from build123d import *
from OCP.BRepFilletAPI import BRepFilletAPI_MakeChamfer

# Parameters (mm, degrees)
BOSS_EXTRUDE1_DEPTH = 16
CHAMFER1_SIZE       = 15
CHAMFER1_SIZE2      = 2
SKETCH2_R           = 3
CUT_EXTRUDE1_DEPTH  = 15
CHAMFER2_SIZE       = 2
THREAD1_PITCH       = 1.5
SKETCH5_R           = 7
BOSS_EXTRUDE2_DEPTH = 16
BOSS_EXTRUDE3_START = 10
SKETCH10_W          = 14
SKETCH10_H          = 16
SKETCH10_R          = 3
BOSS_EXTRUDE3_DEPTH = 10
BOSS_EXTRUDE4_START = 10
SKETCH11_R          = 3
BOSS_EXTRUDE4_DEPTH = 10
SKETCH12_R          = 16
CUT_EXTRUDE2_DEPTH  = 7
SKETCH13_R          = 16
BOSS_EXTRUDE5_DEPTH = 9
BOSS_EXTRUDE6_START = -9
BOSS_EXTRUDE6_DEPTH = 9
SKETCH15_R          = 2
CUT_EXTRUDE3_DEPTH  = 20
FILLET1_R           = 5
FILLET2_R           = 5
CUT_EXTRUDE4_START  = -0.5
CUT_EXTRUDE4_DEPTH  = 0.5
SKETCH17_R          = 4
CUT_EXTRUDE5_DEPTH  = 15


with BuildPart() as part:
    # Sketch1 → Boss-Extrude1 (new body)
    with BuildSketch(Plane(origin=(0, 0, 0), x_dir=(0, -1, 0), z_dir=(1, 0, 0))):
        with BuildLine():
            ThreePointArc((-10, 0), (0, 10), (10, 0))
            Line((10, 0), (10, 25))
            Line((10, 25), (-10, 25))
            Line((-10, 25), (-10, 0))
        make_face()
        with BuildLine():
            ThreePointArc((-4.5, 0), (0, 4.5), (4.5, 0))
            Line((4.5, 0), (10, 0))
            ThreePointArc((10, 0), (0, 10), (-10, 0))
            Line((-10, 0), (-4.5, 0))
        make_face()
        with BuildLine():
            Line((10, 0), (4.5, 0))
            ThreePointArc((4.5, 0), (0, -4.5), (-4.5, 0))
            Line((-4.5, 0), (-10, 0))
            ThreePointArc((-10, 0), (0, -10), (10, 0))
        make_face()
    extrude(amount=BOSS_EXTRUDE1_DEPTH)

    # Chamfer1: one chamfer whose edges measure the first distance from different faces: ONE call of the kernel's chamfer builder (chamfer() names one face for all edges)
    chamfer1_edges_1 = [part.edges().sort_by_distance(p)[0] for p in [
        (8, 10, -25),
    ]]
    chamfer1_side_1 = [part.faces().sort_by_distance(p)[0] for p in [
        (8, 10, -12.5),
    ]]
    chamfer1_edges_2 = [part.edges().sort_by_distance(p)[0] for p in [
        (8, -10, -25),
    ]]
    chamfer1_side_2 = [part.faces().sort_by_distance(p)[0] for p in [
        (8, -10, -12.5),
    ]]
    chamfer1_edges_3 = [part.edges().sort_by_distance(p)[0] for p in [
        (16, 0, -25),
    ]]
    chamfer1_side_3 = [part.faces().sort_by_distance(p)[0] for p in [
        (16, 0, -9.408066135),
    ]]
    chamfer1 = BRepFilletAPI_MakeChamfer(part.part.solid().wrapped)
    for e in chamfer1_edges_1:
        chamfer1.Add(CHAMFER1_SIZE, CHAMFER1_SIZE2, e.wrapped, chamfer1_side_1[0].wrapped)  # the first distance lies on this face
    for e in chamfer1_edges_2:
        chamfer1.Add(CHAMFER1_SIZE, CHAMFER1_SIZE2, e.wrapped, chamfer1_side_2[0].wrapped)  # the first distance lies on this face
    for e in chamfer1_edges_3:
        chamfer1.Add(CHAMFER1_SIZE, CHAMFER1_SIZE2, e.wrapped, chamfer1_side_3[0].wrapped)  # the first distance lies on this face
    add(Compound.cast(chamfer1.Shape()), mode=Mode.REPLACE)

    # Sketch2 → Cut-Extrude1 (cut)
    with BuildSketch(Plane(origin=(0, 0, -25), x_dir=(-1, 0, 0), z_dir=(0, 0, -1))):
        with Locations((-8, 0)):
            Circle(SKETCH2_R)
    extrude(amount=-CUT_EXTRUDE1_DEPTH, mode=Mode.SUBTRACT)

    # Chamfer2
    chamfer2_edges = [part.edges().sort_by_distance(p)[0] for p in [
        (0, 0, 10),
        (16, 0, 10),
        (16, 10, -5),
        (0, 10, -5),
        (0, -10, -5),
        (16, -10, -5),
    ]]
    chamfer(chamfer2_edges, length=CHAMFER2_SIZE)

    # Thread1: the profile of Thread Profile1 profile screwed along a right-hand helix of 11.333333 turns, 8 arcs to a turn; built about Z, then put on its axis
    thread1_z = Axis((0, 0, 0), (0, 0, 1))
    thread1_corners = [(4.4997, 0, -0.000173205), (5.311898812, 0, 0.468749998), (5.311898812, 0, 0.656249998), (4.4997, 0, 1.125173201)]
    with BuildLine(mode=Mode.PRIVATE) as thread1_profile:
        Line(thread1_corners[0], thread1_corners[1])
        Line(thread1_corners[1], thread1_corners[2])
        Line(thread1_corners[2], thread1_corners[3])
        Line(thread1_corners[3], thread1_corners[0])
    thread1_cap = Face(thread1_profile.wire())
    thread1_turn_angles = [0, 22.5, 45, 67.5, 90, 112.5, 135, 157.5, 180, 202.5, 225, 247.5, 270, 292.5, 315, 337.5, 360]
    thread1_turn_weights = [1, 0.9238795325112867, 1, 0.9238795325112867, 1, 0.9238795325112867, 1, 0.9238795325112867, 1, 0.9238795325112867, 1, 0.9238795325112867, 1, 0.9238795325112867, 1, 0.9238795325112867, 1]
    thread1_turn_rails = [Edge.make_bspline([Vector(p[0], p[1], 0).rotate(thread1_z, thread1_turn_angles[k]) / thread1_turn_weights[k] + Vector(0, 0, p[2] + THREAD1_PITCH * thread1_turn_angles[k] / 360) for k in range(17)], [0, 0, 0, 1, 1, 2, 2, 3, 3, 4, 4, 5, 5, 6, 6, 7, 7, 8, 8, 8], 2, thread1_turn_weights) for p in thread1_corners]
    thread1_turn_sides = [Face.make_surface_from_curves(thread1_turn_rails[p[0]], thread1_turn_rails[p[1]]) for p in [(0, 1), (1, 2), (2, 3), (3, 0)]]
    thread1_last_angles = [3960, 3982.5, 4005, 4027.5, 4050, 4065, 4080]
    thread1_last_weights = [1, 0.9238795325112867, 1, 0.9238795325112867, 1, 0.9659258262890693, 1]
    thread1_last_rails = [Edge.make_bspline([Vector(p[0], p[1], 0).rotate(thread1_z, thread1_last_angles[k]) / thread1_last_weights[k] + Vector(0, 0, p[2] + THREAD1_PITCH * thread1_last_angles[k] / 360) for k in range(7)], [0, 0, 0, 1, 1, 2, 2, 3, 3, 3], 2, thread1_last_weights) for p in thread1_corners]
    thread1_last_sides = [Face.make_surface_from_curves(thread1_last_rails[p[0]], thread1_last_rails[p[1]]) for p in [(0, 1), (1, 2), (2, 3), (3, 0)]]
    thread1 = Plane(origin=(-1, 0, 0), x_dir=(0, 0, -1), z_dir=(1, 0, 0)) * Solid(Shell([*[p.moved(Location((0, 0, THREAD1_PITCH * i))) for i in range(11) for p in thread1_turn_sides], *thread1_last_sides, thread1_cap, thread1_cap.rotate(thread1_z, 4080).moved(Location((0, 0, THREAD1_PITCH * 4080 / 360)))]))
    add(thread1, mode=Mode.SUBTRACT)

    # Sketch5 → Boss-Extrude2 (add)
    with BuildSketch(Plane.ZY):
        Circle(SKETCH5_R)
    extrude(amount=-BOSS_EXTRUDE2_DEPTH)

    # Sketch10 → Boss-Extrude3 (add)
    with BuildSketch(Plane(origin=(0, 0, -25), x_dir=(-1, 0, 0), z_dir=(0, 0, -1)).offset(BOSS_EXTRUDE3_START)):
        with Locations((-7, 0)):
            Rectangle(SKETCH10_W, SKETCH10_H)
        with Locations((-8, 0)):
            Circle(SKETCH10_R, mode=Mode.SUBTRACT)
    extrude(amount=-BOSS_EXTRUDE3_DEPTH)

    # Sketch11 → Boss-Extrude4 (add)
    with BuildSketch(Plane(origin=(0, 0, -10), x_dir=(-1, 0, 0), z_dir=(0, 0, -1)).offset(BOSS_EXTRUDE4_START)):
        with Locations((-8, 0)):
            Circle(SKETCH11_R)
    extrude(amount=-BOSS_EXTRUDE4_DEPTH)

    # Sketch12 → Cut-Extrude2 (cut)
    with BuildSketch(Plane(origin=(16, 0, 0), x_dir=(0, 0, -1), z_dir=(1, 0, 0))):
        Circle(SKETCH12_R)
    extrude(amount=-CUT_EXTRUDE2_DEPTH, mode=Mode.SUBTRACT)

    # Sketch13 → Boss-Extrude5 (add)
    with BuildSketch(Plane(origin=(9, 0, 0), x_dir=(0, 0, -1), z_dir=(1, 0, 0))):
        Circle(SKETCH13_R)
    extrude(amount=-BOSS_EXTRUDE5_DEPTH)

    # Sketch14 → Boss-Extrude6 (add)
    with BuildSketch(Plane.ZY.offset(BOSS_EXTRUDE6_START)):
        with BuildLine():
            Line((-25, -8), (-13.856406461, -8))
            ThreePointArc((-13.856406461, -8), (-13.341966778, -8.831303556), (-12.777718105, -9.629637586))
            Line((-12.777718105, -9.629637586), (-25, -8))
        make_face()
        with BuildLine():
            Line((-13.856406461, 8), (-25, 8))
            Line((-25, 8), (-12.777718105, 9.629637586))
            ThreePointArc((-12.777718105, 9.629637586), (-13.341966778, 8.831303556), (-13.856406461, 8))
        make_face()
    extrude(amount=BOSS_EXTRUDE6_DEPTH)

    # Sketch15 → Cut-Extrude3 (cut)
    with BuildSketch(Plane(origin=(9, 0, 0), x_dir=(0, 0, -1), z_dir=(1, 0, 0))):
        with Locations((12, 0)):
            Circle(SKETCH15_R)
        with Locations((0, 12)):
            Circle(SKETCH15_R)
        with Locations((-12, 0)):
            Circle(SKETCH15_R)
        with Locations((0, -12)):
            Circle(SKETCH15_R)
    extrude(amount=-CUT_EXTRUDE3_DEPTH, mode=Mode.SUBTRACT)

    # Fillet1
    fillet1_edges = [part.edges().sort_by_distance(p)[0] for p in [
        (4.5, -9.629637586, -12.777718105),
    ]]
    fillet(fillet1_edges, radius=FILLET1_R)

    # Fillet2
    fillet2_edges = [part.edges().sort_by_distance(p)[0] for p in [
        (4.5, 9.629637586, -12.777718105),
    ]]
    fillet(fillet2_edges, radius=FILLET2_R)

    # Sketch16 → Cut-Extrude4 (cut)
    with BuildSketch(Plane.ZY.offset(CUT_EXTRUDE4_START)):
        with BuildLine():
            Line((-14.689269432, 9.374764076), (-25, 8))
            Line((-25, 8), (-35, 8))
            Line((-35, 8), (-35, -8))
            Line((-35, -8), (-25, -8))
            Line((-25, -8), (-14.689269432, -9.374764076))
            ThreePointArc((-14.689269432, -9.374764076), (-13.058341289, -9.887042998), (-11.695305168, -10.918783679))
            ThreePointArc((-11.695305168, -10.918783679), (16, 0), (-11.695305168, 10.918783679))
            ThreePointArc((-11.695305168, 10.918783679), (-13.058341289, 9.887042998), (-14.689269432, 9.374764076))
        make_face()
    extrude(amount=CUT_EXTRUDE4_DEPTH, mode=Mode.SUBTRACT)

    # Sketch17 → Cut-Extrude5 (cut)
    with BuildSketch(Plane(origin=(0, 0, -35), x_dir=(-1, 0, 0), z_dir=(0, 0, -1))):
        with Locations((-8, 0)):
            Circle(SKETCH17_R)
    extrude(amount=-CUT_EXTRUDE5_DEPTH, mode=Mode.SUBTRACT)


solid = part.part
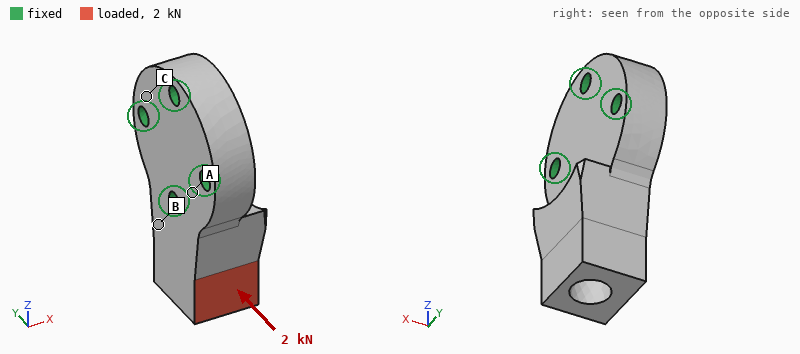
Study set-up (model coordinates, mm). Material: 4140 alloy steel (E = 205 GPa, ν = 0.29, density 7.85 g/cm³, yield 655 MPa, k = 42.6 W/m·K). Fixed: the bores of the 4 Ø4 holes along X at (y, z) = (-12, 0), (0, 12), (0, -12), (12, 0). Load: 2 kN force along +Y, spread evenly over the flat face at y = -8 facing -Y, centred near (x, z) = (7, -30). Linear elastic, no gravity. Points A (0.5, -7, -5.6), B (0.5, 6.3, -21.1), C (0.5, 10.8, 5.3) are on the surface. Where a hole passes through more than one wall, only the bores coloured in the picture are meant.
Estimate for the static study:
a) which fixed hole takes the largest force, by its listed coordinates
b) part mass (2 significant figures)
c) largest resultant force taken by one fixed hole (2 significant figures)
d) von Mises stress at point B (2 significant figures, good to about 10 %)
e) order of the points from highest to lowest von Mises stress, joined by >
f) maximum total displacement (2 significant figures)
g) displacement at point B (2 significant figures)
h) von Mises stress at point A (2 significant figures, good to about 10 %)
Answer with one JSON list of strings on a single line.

["(0, -12)", "81 g", "2.0 kN", "35 MPa", "B > A > C", "15 µm", "4.2 µm", "19 MPa"]
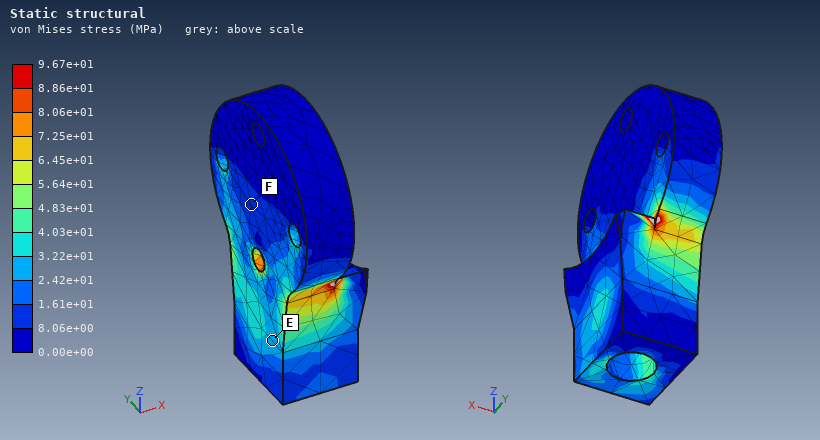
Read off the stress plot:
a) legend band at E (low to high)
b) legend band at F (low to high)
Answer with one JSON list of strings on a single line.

["2.42e+01 to 3.22e+01 MPa", "8.06e+00 to 1.61e+01 MPa"]
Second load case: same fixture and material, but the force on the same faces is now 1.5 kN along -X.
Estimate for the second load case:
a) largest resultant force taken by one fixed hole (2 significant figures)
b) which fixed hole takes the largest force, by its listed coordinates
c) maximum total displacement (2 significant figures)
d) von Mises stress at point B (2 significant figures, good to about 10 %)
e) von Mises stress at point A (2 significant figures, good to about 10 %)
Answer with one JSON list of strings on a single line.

["2.1 kN", "(0, -12)", "28 µm", "46 MPa", "22 MPa"]
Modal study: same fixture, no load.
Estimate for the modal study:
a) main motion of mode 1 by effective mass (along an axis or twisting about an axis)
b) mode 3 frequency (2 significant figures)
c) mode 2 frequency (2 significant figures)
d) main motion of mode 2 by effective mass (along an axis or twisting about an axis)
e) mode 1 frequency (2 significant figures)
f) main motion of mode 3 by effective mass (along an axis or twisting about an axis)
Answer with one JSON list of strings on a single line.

["along X", "24 kHz", "17 kHz", "along Y", "11 kHz", "twisting about Z"]
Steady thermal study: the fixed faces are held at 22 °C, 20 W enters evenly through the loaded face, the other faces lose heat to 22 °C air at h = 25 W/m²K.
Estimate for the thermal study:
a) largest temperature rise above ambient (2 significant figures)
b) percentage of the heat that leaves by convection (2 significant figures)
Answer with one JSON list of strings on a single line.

["71 K", "7.7 %"]
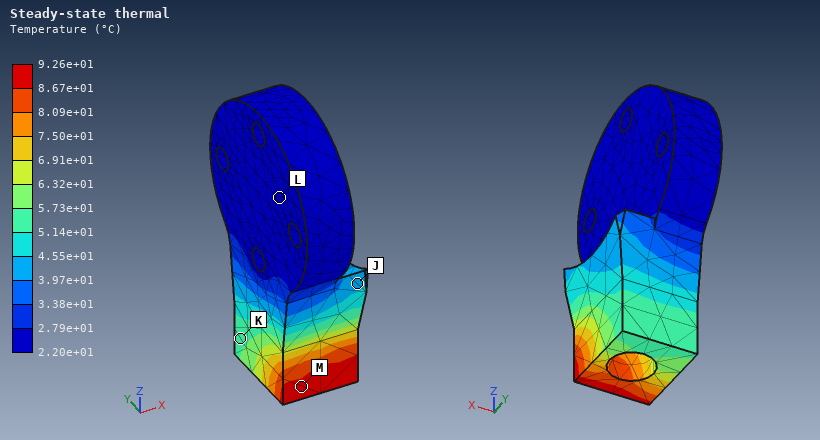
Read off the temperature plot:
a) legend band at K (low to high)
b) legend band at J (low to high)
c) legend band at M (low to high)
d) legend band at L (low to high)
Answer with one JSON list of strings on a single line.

["5.14e+01 to 5.73e+01 °C", "3.97e+01 to 4.55e+01 °C", "8.67e+01 to 9.26e+01 °C", "2.20e+01 to 2.79e+01 °C"]
